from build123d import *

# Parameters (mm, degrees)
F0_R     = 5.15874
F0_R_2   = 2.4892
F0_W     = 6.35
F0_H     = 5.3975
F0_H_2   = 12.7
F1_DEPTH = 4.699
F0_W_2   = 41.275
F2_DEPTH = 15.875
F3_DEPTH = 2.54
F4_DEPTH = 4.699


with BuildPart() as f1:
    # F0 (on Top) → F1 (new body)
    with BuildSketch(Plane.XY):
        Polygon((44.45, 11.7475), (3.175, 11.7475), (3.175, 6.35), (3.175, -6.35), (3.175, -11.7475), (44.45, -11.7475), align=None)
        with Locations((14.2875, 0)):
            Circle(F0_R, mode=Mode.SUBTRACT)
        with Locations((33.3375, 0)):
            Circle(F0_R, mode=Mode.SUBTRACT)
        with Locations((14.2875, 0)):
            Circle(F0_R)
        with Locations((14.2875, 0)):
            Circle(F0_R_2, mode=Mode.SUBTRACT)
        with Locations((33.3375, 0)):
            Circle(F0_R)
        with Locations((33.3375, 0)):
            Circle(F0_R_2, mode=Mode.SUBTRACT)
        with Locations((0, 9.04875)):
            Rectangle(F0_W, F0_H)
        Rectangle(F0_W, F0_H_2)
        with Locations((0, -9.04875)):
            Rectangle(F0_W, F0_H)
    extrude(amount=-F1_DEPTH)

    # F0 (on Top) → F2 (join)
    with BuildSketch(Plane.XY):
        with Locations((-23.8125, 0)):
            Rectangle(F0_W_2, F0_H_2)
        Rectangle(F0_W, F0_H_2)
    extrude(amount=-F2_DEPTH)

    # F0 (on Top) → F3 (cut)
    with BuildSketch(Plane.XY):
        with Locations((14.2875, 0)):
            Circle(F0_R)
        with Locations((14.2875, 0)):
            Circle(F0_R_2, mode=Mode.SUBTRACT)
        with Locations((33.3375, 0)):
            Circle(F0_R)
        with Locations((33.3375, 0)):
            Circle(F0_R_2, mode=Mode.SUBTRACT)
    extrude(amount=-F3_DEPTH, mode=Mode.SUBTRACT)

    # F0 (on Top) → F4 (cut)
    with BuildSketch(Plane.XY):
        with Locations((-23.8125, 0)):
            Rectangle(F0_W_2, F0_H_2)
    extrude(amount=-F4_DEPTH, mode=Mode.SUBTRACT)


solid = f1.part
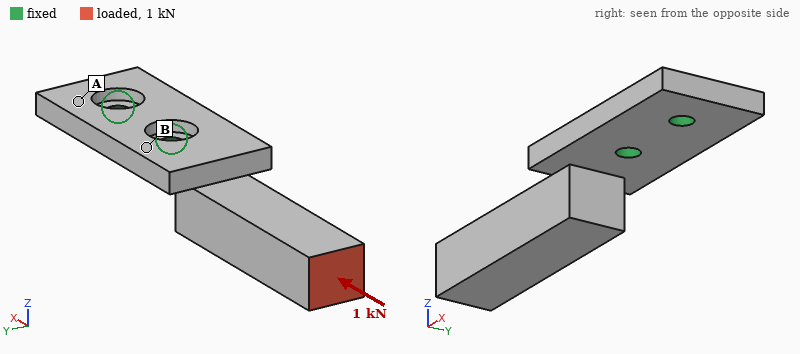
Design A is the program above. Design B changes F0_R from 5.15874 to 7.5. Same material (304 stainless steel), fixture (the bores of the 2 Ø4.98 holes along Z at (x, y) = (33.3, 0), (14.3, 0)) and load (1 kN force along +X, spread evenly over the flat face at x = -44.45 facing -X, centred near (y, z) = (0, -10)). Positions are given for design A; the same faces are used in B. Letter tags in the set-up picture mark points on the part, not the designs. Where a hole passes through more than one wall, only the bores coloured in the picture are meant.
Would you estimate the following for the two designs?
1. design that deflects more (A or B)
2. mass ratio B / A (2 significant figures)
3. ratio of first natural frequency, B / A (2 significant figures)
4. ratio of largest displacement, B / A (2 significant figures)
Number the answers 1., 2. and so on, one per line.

1. B
2. 0.96
3. 0.89
4. 1.2
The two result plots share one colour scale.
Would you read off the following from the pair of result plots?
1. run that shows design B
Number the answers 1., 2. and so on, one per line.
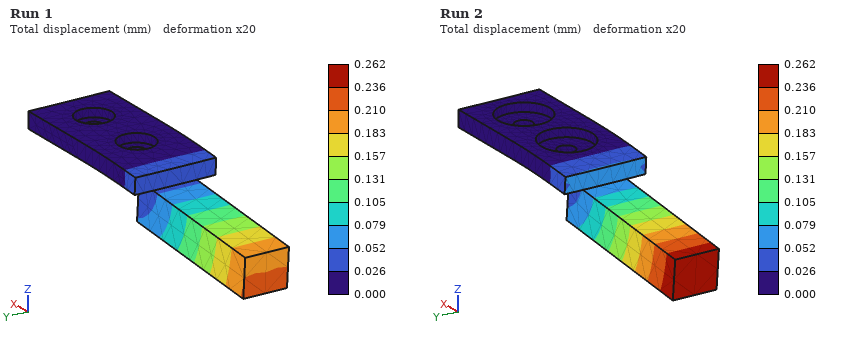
1. Run 2
